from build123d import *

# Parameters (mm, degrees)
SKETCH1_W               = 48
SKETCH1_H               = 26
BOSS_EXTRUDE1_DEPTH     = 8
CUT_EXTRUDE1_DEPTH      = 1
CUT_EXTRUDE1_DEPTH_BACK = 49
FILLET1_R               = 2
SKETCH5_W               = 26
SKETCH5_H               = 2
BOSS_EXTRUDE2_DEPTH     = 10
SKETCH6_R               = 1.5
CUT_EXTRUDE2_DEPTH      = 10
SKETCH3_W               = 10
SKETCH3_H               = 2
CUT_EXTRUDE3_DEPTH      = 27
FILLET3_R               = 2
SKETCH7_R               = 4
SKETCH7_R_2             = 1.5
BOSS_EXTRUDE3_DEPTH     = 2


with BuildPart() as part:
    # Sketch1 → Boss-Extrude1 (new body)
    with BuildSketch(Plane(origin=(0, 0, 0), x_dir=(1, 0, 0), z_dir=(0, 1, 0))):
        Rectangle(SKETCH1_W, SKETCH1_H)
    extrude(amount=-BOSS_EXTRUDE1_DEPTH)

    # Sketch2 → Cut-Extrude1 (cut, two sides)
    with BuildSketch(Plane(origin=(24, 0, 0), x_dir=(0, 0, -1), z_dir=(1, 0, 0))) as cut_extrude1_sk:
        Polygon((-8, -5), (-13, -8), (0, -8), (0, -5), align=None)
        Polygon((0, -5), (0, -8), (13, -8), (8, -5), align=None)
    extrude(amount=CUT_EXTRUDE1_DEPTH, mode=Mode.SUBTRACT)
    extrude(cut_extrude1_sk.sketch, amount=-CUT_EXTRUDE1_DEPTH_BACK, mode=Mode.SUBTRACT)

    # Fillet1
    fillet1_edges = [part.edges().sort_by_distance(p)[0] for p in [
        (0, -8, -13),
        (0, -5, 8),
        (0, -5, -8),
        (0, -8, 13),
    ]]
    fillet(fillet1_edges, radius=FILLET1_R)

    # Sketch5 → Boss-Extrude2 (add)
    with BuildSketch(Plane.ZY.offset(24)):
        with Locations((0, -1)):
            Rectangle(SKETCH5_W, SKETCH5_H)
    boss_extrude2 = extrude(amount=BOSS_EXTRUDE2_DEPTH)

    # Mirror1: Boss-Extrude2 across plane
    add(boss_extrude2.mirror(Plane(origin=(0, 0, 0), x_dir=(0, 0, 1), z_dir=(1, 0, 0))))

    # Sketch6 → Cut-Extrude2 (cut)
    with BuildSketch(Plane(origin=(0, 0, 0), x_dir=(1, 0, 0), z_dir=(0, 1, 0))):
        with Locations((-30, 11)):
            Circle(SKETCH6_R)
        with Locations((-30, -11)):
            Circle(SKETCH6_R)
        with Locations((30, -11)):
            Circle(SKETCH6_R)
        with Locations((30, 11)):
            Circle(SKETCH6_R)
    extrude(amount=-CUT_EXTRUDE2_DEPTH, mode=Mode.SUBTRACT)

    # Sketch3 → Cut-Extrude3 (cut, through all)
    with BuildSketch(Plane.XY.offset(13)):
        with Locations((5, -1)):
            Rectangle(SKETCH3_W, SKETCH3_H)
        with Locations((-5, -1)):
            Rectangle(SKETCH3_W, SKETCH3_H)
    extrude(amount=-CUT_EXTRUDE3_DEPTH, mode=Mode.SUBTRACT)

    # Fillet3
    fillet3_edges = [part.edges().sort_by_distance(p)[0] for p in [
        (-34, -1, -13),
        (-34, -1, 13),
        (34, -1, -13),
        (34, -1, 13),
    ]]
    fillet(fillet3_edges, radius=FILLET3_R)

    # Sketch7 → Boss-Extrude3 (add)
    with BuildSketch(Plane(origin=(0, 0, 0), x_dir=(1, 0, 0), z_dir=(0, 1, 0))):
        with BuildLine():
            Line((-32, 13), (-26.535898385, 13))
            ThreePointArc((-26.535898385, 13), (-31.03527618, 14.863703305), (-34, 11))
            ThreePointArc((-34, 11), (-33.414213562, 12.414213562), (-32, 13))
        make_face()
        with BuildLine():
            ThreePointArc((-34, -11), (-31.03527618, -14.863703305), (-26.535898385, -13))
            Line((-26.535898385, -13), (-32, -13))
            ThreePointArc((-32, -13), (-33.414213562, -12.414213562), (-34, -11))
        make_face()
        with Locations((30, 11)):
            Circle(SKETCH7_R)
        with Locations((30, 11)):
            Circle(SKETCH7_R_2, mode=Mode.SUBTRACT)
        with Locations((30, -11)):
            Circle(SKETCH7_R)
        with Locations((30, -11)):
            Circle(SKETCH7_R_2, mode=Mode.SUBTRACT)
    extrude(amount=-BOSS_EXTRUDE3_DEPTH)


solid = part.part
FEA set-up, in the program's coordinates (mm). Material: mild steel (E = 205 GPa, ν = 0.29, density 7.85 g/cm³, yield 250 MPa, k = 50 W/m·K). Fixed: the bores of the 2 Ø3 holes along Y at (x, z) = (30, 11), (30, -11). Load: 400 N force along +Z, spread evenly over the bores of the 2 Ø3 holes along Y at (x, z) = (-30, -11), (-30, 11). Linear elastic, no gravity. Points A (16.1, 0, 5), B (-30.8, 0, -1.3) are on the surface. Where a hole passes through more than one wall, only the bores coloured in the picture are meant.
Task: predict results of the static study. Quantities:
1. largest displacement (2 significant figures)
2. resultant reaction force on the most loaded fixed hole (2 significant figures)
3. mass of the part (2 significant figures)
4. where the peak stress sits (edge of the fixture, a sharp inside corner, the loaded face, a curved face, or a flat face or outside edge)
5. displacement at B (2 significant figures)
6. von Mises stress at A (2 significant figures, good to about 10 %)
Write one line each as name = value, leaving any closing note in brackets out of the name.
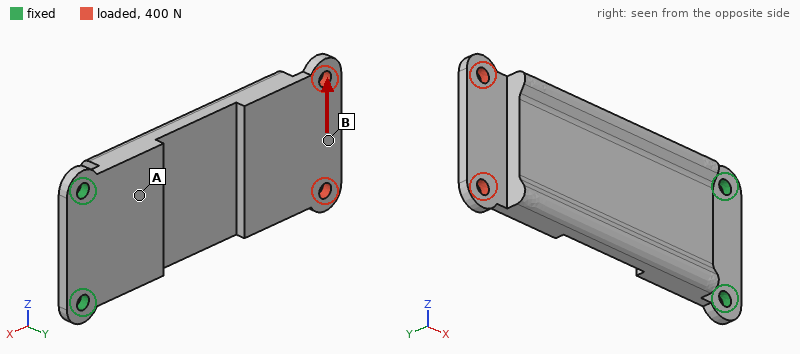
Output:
largest displacement = 55 µm
resultant reaction force on the most loaded fixed hole = 1.1 kN
mass of the part = 53 g
where the peak stress sits = a flat face or outside edge
displacement at B = 46 µm
von Mises stress at A = 46 MPa
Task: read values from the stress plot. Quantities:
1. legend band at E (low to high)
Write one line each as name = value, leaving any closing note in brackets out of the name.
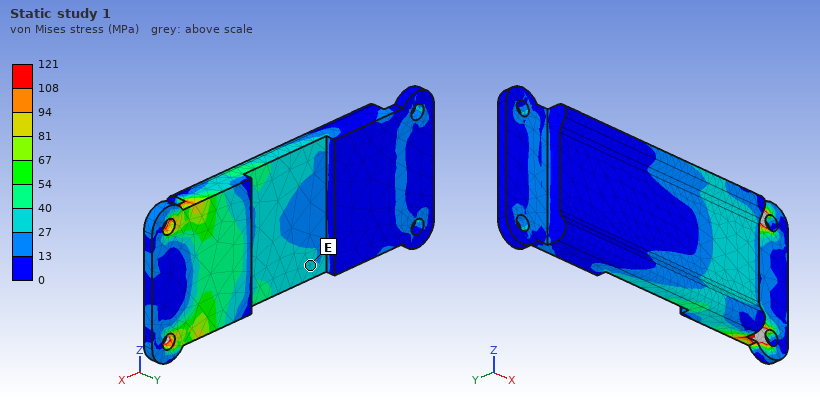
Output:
legend band at E = 27 to 40 MPa
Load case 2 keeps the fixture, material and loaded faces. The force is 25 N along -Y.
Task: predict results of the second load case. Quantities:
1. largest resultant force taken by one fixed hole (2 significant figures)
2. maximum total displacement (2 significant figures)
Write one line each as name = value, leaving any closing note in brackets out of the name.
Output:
largest resultant force taken by one fixed hole = 15 N
maximum total displacement = 0.21 mm
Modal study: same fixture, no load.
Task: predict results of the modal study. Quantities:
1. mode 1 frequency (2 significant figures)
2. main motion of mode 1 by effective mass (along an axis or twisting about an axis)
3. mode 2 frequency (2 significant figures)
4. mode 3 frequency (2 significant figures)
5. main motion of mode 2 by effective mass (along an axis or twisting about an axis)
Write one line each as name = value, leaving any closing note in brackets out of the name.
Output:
mode 1 frequency = 460 Hz
main motion of mode 1 by effective mass = along Y
mode 2 frequency = 3400 Hz
mode 3 frequency = 4000 Hz
main motion of mode 2 by effective mass = along Z
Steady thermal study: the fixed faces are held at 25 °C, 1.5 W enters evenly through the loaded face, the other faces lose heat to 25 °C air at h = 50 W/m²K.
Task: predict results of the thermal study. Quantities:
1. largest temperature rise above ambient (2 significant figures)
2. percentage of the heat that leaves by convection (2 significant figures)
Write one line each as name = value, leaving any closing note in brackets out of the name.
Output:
largest temperature rise above ambient = 14 K
percentage of the heat that leaves by convection = 70 %
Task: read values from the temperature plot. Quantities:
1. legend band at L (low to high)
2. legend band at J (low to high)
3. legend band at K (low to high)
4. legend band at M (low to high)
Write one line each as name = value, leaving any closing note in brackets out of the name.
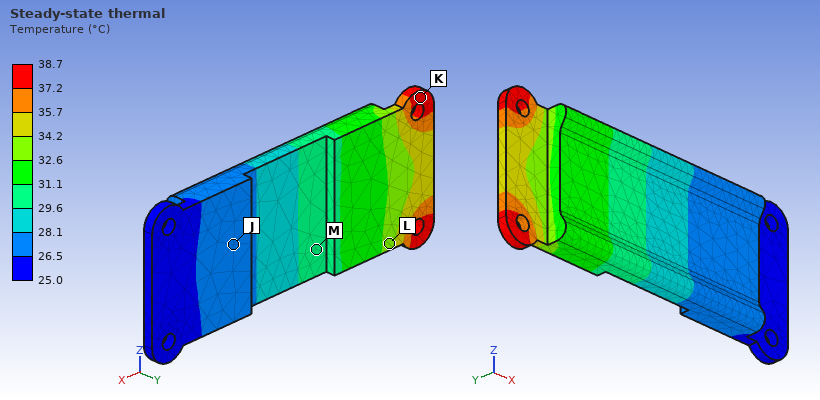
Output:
legend band at L = 32.6 to 34.2 °C
legend band at J = 26.5 to 28.1 °C
legend band at K = 37.2 to 38.7 °C
legend band at M = 29.6 to 31.1 °C
